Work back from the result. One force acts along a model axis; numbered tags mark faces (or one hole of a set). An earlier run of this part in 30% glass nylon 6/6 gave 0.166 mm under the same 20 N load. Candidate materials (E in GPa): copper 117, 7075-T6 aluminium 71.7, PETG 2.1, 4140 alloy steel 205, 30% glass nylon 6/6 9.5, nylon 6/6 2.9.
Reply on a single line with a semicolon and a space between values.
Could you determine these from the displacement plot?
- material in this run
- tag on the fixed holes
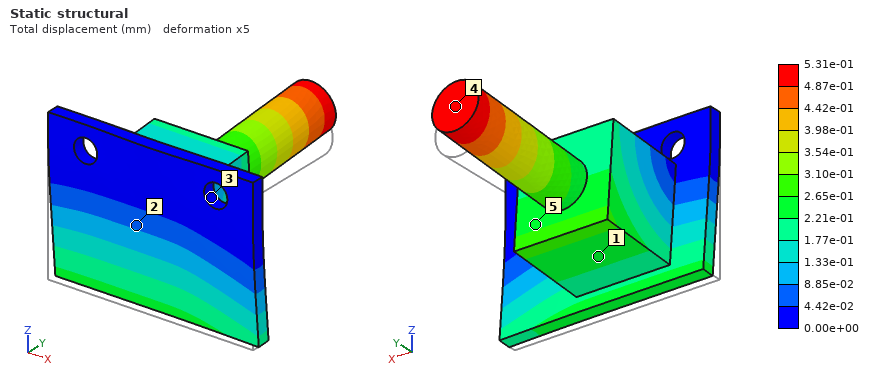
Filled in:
nylon 6/6; 3
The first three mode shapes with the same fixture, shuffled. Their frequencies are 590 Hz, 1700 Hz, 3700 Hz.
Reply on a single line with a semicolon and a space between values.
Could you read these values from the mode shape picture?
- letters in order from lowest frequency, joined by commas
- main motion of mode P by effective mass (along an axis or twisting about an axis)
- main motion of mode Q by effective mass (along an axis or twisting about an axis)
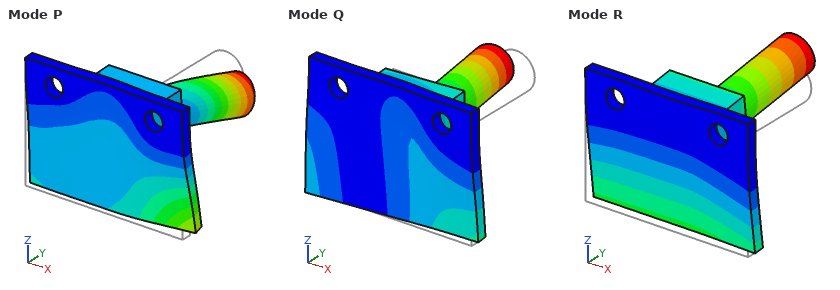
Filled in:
R, Q, P; along Y; along X
